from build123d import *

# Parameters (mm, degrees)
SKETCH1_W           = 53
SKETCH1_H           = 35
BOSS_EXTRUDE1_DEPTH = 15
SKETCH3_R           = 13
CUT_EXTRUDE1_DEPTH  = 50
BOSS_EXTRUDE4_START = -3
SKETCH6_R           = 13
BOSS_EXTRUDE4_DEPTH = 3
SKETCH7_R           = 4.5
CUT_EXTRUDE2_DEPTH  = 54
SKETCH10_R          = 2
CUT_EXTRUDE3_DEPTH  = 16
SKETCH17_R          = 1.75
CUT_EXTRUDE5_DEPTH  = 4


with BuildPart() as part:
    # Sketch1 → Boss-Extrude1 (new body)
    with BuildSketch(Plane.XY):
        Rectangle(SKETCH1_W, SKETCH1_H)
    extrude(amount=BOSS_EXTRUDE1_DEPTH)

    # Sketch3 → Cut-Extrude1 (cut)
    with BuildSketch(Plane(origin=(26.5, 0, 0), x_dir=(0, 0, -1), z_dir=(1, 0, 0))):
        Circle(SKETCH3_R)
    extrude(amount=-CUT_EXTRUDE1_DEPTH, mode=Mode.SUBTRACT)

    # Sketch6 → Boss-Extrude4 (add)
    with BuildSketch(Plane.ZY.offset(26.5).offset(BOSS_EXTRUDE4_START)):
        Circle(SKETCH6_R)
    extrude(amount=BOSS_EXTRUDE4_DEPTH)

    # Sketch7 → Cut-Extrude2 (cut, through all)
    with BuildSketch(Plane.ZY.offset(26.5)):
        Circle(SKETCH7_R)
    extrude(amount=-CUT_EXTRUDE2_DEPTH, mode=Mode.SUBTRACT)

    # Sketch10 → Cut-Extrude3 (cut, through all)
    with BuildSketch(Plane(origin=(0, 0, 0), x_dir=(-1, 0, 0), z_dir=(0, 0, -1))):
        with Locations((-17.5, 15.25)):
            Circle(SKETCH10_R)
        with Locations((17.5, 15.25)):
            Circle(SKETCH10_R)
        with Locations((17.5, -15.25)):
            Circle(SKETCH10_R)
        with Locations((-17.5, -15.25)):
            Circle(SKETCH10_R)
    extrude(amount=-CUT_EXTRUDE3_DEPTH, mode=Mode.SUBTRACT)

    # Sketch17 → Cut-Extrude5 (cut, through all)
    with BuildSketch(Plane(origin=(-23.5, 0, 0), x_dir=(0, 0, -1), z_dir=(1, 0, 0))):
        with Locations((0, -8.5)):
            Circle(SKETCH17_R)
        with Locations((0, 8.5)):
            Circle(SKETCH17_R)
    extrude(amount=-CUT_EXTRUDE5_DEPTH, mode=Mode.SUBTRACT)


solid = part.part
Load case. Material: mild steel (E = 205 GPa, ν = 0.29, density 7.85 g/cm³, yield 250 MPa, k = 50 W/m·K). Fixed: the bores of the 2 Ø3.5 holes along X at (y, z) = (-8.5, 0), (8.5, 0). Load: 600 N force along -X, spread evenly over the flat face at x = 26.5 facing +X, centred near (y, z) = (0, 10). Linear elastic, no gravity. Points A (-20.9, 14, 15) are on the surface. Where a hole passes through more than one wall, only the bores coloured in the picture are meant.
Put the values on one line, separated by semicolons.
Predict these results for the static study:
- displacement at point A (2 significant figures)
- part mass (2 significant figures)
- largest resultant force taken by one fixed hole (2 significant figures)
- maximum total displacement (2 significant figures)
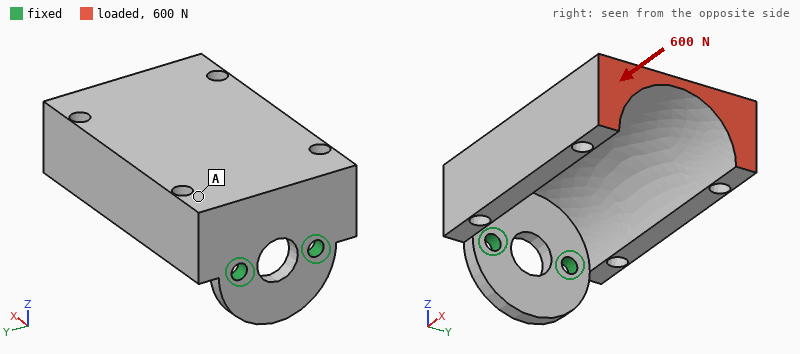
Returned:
22 µm; 110 g; 300 N; 80 µm
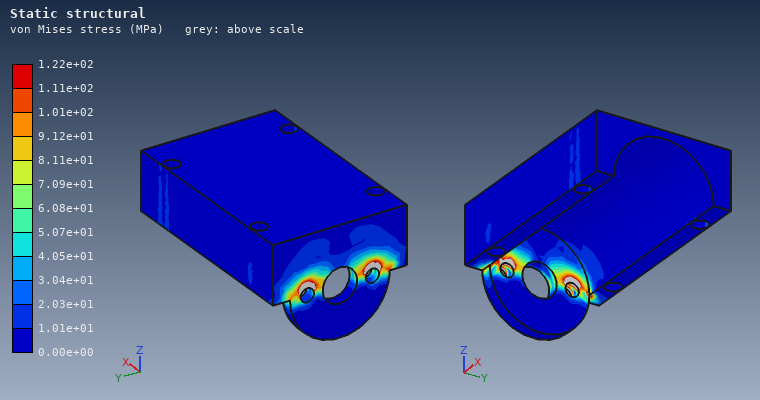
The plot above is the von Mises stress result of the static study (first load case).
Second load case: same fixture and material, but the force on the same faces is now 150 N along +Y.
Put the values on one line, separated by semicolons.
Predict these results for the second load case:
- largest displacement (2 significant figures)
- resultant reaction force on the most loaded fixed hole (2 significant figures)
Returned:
35 µm; 340 N
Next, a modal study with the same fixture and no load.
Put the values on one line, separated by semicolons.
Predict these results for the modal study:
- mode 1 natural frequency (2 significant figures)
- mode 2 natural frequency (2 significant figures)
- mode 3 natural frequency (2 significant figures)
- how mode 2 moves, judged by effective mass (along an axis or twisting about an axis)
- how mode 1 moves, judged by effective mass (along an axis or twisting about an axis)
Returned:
840 Hz; 1800 Hz; 4500 Hz; along Y; along Z
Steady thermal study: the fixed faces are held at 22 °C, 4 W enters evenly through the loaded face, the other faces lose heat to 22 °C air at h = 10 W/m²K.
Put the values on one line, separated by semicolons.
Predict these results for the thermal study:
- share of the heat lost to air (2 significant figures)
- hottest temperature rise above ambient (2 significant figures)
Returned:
23 %; 22 K
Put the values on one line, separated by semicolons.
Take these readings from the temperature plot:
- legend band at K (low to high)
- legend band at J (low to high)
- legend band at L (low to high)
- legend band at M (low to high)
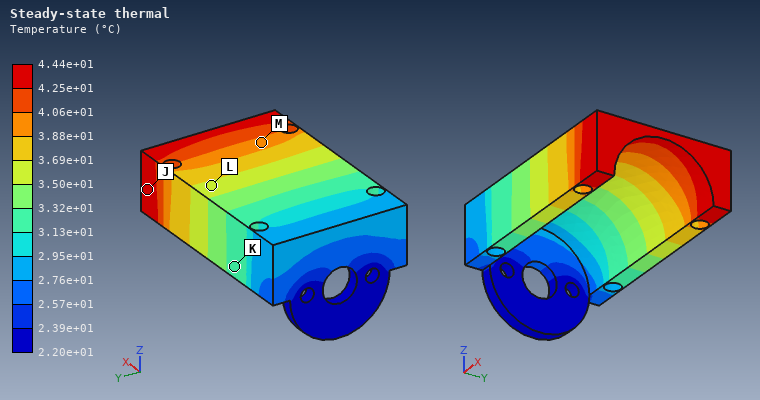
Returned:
3.13e+01 to 3.32e+01 °C; 4.25e+01 to 4.44e+01 °C; 3.50e+01 to 3.69e+01 °C; 3.88e+01 to 4.06e+01 °C
